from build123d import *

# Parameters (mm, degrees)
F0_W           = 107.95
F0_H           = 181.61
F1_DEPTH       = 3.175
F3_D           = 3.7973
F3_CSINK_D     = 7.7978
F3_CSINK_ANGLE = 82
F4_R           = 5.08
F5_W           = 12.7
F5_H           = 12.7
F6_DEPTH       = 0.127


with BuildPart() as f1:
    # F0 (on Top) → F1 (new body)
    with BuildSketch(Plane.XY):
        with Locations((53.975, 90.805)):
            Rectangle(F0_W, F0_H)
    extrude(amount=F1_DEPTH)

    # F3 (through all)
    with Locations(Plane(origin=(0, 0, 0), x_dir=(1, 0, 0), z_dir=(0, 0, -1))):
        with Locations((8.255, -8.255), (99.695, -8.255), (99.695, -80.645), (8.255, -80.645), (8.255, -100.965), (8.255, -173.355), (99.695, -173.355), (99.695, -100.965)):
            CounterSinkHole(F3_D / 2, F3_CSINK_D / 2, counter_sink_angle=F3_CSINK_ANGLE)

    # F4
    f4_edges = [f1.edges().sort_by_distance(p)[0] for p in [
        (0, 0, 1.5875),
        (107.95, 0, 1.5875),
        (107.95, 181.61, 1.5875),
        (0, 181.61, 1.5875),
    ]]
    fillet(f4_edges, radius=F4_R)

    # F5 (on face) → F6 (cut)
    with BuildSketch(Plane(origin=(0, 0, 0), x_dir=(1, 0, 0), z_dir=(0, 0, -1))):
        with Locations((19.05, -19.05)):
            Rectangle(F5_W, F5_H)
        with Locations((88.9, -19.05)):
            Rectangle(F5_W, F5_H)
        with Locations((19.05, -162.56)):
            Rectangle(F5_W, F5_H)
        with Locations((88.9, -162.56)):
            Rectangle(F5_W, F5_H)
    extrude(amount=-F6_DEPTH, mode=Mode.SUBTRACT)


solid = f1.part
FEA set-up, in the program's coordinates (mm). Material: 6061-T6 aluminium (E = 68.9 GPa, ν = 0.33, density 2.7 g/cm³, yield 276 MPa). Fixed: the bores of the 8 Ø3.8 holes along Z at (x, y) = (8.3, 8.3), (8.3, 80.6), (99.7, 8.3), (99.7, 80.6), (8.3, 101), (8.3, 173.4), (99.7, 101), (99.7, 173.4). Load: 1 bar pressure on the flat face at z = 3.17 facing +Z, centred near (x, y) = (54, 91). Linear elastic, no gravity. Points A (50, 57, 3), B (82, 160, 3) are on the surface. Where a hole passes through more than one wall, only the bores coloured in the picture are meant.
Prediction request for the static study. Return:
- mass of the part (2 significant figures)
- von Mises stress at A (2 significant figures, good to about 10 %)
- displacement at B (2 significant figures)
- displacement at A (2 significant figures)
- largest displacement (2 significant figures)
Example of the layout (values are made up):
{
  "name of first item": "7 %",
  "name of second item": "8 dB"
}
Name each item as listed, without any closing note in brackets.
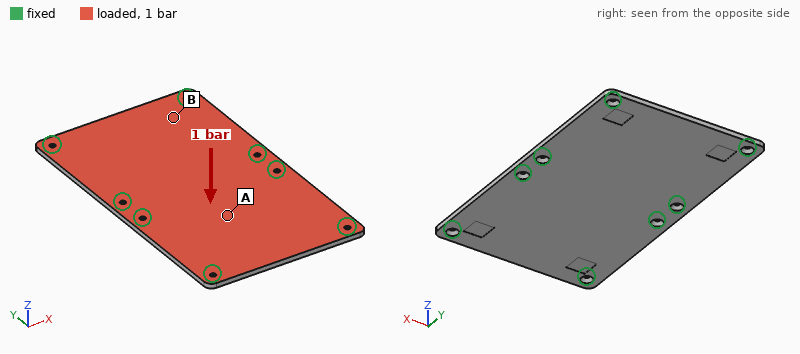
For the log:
{
  "mass of the part": "170 g",
  "von Mises stress at A": "24 MPa",
  "displacement at B": "0.13 mm",
  "displacement at A": "0.23 mm",
  "largest displacement": "0.24 mm"
}
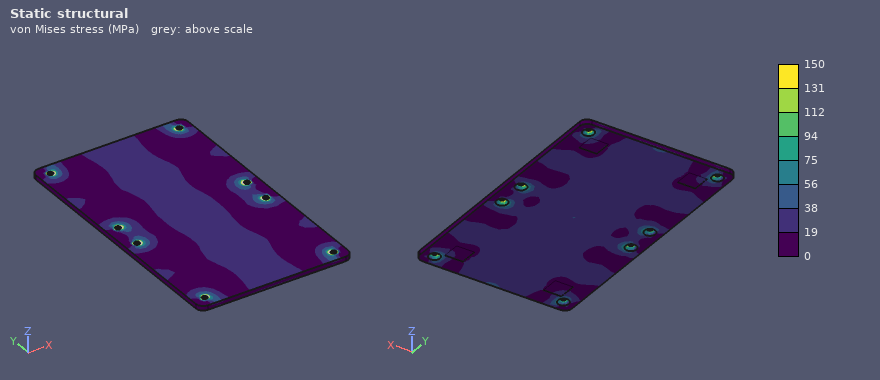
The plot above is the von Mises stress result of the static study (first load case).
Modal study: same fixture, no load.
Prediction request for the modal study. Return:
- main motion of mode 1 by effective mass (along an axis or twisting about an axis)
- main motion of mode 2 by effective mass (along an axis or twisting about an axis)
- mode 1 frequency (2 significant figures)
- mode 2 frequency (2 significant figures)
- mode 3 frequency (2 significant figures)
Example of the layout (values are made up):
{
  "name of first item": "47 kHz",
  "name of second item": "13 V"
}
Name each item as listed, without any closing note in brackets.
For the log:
{
  "main motion of mode 1 by effective mass": "along Z",
  "main motion of mode 2 by effective mass": "twisting about X",
  "mode 1 frequency": "1300 Hz",
  "mode 2 frequency": "1400 Hz",
  "mode 3 frequency": "2100 Hz"
}
